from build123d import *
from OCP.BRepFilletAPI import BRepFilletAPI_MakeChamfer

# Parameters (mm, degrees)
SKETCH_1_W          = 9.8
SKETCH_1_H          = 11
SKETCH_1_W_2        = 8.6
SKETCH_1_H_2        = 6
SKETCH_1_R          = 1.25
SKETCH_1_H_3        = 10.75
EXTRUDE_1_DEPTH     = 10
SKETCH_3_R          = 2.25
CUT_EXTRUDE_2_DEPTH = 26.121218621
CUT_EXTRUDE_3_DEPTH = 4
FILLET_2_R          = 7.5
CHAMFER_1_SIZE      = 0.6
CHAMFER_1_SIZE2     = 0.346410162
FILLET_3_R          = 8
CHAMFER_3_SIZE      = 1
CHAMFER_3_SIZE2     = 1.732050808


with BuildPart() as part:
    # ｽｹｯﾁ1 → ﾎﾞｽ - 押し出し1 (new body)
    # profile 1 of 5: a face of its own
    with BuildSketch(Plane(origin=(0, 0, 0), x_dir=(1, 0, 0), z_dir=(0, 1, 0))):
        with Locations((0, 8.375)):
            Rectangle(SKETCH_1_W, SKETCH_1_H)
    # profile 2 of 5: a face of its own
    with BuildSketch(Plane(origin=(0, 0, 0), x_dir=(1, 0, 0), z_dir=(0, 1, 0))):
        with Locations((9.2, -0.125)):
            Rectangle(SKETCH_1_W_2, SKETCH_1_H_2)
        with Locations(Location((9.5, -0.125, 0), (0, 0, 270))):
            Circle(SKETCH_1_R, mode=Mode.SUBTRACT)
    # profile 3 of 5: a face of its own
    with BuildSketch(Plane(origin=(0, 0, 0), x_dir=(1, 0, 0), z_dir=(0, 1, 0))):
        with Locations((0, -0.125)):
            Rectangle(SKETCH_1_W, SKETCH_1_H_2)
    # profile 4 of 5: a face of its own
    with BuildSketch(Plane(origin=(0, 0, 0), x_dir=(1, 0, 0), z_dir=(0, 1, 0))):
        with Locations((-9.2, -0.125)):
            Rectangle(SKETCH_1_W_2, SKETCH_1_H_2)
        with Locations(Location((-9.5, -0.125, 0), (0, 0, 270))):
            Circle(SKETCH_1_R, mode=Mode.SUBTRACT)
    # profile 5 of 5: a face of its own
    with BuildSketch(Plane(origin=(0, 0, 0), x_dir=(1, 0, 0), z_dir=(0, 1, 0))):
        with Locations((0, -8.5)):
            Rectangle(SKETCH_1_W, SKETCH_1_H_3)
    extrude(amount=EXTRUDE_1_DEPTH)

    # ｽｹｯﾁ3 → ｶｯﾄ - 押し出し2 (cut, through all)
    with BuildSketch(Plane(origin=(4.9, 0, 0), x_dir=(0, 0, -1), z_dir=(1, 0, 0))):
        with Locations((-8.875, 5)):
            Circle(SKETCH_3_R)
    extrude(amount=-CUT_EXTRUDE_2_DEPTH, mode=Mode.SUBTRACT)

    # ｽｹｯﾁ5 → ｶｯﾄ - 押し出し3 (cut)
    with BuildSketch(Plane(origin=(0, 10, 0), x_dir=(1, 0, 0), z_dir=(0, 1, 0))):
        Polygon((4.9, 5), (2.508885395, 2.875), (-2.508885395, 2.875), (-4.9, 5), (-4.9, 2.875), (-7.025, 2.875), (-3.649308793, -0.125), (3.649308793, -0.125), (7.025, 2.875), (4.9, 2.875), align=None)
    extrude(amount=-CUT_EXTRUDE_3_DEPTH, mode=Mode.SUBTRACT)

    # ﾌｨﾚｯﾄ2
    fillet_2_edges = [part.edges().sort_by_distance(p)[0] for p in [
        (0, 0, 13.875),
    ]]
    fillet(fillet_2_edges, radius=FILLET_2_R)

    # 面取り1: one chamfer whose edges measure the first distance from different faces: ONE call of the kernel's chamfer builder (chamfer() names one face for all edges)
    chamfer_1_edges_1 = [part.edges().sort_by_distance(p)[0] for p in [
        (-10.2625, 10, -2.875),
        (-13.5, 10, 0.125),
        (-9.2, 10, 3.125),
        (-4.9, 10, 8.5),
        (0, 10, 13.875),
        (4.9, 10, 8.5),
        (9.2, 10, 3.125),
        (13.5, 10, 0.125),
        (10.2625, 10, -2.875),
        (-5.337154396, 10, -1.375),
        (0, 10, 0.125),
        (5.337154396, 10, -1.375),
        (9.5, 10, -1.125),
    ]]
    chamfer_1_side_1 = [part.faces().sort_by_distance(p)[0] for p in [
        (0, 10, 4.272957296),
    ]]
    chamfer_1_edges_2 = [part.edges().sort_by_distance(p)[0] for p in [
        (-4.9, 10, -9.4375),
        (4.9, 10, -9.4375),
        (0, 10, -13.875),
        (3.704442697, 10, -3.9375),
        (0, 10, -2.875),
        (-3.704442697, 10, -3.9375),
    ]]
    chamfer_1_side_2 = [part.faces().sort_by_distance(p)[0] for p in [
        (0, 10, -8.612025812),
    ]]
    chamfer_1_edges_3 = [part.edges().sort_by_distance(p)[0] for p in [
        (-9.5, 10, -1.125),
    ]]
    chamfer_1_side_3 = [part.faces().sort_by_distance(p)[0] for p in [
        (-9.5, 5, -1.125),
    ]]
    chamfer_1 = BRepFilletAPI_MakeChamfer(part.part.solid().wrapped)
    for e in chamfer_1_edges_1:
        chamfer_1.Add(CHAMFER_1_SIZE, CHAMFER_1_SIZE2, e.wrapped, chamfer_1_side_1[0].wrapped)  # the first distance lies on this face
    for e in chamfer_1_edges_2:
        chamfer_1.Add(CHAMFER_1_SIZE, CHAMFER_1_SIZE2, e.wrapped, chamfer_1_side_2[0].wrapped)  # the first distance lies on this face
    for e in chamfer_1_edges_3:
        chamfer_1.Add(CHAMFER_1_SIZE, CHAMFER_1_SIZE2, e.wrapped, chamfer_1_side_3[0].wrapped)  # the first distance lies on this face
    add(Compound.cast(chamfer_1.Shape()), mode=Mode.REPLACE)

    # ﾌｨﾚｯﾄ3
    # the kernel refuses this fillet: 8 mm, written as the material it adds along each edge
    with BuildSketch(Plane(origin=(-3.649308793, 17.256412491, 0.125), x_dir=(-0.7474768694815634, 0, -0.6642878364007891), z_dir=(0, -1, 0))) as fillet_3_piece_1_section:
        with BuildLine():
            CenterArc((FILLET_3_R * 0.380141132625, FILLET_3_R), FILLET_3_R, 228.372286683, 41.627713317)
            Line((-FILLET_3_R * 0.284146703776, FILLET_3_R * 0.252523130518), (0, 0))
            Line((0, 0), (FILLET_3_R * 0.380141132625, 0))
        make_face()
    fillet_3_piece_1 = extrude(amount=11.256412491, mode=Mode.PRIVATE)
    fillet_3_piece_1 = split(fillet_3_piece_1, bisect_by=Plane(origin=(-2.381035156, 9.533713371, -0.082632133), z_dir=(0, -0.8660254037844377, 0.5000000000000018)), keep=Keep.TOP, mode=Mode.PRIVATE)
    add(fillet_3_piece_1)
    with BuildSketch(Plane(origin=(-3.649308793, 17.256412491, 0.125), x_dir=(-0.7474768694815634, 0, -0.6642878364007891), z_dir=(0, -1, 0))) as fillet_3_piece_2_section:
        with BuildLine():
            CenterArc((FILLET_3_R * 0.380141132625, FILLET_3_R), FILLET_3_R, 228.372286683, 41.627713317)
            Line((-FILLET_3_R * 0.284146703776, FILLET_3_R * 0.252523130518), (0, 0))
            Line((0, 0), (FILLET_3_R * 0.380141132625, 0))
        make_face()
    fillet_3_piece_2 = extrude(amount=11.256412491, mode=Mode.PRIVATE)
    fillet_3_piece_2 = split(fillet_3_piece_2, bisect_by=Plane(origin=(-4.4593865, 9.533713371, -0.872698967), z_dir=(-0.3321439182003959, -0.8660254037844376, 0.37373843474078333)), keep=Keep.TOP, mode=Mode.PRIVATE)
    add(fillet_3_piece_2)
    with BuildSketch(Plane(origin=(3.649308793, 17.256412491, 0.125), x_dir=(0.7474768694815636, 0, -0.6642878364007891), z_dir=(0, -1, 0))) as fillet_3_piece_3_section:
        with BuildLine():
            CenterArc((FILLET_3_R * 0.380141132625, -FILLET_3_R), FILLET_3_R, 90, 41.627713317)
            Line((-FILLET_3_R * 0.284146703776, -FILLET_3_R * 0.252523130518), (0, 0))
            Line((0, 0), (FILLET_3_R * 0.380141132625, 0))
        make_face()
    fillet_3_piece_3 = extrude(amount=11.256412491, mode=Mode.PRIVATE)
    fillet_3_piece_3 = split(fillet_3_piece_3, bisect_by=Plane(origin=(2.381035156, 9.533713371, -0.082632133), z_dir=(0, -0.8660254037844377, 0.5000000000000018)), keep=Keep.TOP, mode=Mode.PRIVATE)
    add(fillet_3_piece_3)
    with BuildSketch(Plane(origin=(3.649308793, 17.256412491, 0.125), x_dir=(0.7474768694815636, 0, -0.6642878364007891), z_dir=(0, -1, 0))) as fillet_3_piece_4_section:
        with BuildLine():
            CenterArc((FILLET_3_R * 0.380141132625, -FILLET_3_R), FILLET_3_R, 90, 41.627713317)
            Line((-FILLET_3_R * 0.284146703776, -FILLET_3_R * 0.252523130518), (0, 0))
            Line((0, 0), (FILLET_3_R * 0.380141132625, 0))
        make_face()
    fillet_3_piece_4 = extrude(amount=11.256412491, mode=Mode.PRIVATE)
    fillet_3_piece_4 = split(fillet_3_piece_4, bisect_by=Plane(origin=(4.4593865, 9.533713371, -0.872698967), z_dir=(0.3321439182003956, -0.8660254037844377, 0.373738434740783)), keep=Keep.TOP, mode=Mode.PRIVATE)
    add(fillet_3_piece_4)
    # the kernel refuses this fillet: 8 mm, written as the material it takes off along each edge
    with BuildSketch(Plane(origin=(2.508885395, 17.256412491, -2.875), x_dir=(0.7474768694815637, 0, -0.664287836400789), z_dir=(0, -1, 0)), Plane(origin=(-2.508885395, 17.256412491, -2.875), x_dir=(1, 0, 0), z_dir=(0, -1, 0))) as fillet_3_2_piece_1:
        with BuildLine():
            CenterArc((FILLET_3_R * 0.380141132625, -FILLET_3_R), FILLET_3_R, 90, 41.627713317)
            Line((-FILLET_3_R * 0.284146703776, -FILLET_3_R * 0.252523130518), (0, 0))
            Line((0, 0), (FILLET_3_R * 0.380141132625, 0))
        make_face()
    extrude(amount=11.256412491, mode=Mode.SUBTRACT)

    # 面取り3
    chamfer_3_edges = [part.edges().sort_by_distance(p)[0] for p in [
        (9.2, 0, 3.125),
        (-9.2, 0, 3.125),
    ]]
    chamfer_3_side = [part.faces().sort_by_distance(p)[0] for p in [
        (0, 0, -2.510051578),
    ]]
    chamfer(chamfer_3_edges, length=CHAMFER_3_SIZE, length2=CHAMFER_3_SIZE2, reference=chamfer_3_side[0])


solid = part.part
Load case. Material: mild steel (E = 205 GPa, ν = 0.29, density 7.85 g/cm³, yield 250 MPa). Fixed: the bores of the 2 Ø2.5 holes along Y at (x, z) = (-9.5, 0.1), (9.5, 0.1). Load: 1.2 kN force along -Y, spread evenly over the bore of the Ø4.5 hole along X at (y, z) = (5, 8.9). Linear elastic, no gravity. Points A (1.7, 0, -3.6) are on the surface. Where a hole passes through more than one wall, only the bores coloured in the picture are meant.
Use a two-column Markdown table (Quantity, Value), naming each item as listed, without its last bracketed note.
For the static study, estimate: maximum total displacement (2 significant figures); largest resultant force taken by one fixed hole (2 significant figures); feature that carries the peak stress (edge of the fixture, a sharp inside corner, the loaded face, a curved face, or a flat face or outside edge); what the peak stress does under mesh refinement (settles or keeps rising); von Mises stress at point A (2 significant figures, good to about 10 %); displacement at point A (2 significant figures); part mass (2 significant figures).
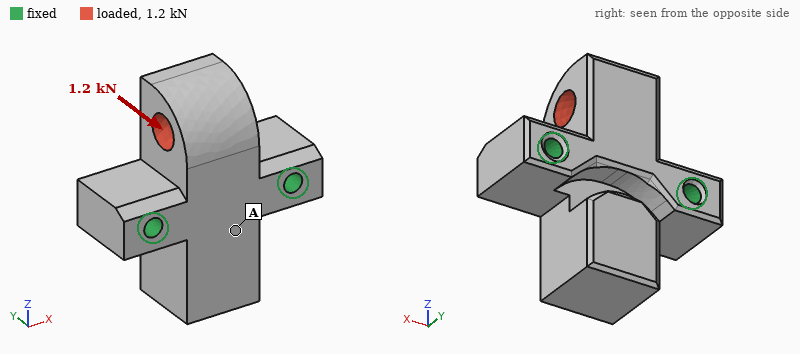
| Quantity | Value |
|---|---|
| maximum total displacement | 16 µm |
| largest resultant force taken by one fixed hole | 650 N |
| feature that carries the peak stress | edge of the fixture |
| what the peak stress does under mesh refinement | keeps rising |
| von Mises stress at point A | 20 MPa |
| displacement at point A | 3.2 µm |
| part mass | 25 g |
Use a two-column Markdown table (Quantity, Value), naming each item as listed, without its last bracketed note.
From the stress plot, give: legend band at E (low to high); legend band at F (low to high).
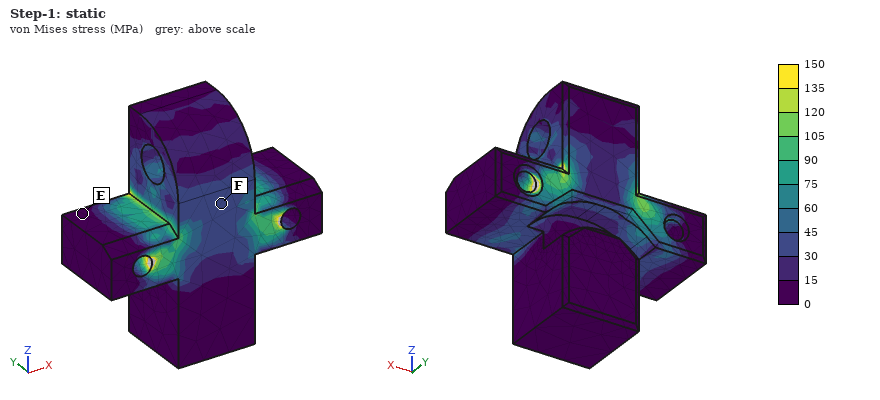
| Quantity | Value |
|---|---|
| legend band at E | 0 to 15 MPa |
| legend band at F | 30 to 45 MPa |
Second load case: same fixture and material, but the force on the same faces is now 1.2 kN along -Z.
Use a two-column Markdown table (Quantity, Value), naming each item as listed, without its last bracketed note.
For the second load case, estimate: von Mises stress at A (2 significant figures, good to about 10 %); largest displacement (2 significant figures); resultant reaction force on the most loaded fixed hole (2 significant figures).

| Quantity | Value |
|---|---|
| von Mises stress at A | 11 MPa |
| largest displacement | 2.3 µm |
| resultant reaction force on the most loaded fixed hole | 630 N |
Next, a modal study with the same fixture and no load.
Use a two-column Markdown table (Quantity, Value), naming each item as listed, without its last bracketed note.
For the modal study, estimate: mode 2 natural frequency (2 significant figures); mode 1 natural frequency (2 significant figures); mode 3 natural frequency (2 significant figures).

| Quantity | Value |
|---|---|
| mode 2 natural frequency | 24 kHz |
| mode 1 natural frequency | 13 kHz |
| mode 3 natural frequency | 24 kHz |
